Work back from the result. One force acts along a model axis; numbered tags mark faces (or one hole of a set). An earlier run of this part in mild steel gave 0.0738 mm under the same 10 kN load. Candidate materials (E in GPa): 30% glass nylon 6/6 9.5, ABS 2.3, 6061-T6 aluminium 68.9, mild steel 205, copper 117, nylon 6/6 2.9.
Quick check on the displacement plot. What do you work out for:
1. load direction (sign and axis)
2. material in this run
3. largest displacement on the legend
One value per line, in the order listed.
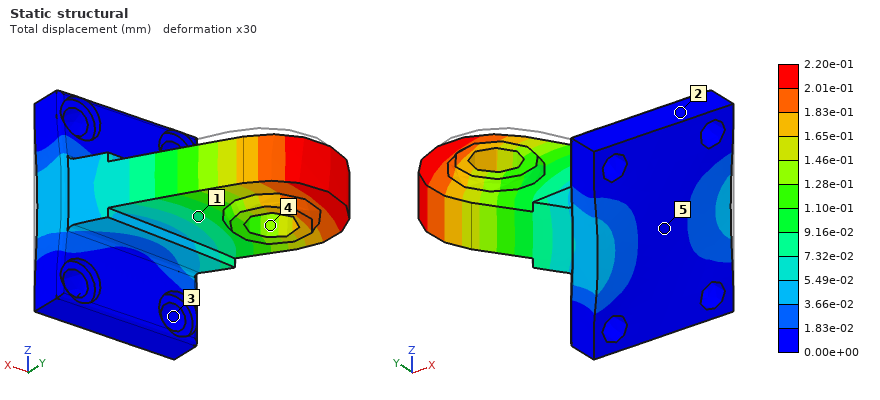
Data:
-X
6061-T6 aluminium
2.20e-01 mm
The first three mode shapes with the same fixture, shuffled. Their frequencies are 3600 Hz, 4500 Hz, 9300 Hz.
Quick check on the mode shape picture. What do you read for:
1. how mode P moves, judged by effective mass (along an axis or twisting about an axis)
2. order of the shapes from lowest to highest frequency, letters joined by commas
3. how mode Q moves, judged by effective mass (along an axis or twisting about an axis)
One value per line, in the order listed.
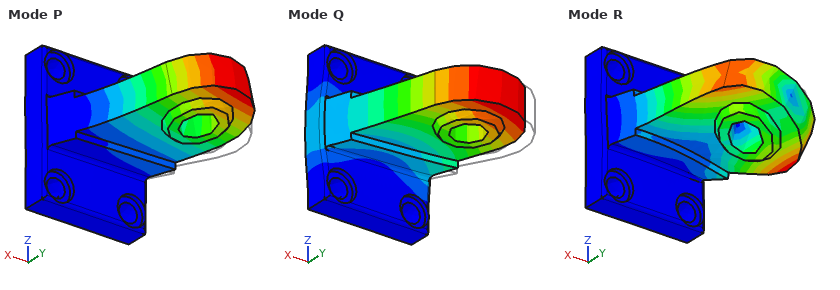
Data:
along Z
P, Q, R
along X
